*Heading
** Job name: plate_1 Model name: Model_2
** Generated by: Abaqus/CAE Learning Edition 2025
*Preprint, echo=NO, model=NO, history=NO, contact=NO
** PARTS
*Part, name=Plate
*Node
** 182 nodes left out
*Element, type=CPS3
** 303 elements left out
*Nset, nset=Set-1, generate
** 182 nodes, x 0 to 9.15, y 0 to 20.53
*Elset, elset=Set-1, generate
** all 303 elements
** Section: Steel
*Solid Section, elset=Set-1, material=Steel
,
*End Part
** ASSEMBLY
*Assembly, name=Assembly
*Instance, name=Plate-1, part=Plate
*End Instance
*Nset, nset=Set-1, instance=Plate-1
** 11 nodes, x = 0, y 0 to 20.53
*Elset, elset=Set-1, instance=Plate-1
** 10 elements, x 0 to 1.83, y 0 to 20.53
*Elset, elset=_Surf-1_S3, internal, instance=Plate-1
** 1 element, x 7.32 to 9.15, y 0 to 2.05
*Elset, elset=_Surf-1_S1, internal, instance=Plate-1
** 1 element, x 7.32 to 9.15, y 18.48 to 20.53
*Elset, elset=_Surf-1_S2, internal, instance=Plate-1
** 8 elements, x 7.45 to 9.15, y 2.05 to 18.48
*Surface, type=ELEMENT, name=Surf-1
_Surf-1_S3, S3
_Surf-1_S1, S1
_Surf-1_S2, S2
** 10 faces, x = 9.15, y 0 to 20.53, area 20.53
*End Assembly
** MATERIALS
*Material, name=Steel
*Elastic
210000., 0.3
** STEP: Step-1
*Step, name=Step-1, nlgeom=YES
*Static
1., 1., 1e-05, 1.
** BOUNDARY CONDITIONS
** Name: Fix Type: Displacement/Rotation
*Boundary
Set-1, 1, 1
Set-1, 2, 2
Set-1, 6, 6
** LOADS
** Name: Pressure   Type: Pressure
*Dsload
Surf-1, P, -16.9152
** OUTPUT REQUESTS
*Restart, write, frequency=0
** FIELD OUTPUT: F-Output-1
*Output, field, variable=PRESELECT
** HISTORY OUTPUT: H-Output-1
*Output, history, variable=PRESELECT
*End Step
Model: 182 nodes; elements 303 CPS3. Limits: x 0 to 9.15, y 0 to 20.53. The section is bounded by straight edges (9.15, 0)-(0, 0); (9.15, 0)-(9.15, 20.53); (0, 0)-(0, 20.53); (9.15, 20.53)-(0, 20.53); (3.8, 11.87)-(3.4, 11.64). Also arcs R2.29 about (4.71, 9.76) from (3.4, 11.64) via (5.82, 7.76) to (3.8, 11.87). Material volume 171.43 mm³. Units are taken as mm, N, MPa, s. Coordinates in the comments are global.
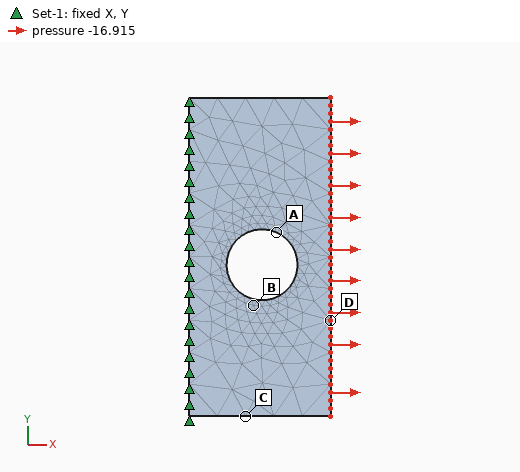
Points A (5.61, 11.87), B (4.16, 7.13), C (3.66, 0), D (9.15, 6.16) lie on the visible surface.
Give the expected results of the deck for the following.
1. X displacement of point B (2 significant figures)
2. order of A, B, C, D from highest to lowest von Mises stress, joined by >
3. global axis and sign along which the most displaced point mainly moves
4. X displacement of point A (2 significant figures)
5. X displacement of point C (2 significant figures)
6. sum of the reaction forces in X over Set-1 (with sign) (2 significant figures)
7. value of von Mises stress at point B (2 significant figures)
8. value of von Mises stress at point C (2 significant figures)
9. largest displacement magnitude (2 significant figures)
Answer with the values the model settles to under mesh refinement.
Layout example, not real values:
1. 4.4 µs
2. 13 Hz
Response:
1. 4.1e-04 mm
2. A > B > D > C
3. +X
4. 7.7e-04 mm
5. 3.5e-04 mm
6. -350 N
7. 35 MPa
8. 14 MPa
9. 0.0014 mm
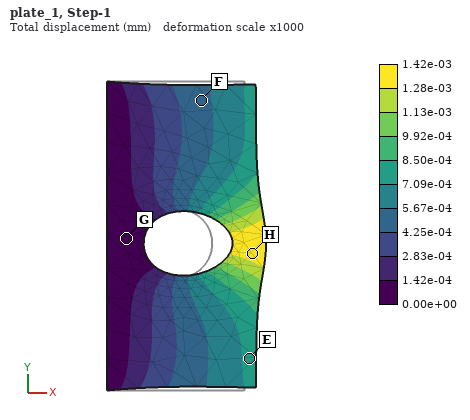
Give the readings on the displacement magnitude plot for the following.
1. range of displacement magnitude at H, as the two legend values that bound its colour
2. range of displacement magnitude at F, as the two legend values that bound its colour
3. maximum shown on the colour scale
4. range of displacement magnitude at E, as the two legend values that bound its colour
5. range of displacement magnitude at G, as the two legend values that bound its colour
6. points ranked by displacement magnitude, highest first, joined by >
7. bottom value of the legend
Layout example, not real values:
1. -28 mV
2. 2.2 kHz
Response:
1. 1.28e-03 to 1.42e-03 mm
2. 4.25e-04 to 5.67e-04 mm
3. 1.42e-03 mm
4. 7.09e-04 to 8.50e-04 mm
5. 0.00e+00 to 1.42e-04 mm
6. H > E > F > G
7. 0.00e+00 mm
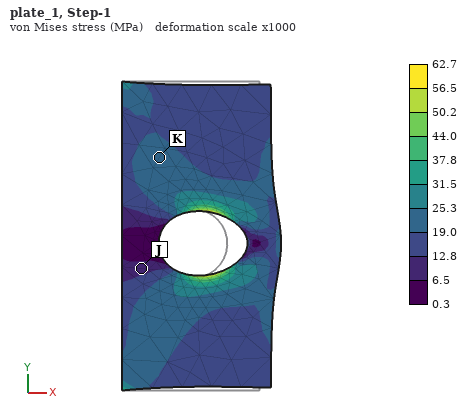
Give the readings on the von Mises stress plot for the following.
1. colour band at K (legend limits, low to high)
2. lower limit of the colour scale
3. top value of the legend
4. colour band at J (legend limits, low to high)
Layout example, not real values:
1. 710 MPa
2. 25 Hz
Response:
1. 19.0 to 25.3 MPa
2. 0.3 MPa
3. 62.7 MPa
4. 6.5 to 12.8 MPa
